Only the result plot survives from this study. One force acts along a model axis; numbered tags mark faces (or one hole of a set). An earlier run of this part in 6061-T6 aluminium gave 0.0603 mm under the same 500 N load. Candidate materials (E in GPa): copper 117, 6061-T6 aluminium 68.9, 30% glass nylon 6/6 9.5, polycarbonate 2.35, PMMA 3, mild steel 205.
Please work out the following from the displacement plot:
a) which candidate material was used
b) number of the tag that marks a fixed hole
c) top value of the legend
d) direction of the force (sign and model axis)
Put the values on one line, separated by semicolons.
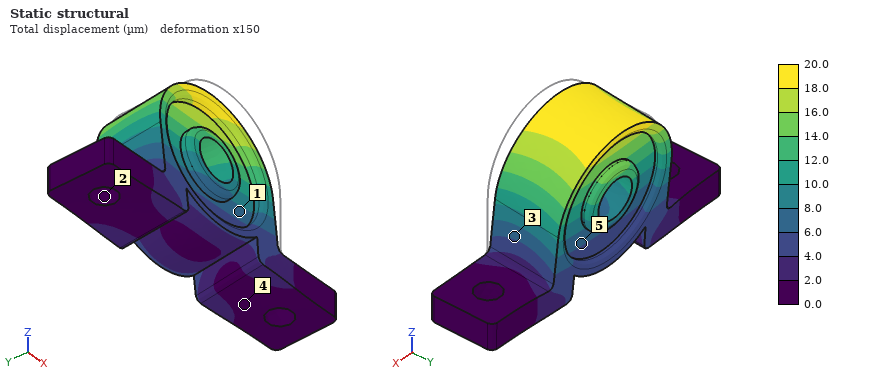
mild steel; 2; 20.0 µm; +Y
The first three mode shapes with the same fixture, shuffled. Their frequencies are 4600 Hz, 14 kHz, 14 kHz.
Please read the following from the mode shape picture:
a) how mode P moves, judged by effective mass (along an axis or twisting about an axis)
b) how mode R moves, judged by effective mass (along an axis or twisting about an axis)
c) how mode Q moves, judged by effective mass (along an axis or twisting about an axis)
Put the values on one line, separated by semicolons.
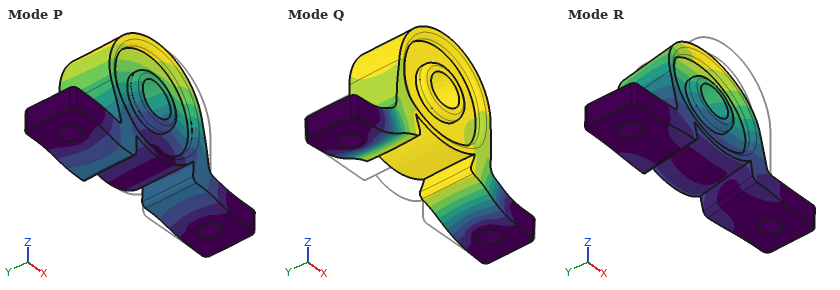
along X; along Y; along Z
